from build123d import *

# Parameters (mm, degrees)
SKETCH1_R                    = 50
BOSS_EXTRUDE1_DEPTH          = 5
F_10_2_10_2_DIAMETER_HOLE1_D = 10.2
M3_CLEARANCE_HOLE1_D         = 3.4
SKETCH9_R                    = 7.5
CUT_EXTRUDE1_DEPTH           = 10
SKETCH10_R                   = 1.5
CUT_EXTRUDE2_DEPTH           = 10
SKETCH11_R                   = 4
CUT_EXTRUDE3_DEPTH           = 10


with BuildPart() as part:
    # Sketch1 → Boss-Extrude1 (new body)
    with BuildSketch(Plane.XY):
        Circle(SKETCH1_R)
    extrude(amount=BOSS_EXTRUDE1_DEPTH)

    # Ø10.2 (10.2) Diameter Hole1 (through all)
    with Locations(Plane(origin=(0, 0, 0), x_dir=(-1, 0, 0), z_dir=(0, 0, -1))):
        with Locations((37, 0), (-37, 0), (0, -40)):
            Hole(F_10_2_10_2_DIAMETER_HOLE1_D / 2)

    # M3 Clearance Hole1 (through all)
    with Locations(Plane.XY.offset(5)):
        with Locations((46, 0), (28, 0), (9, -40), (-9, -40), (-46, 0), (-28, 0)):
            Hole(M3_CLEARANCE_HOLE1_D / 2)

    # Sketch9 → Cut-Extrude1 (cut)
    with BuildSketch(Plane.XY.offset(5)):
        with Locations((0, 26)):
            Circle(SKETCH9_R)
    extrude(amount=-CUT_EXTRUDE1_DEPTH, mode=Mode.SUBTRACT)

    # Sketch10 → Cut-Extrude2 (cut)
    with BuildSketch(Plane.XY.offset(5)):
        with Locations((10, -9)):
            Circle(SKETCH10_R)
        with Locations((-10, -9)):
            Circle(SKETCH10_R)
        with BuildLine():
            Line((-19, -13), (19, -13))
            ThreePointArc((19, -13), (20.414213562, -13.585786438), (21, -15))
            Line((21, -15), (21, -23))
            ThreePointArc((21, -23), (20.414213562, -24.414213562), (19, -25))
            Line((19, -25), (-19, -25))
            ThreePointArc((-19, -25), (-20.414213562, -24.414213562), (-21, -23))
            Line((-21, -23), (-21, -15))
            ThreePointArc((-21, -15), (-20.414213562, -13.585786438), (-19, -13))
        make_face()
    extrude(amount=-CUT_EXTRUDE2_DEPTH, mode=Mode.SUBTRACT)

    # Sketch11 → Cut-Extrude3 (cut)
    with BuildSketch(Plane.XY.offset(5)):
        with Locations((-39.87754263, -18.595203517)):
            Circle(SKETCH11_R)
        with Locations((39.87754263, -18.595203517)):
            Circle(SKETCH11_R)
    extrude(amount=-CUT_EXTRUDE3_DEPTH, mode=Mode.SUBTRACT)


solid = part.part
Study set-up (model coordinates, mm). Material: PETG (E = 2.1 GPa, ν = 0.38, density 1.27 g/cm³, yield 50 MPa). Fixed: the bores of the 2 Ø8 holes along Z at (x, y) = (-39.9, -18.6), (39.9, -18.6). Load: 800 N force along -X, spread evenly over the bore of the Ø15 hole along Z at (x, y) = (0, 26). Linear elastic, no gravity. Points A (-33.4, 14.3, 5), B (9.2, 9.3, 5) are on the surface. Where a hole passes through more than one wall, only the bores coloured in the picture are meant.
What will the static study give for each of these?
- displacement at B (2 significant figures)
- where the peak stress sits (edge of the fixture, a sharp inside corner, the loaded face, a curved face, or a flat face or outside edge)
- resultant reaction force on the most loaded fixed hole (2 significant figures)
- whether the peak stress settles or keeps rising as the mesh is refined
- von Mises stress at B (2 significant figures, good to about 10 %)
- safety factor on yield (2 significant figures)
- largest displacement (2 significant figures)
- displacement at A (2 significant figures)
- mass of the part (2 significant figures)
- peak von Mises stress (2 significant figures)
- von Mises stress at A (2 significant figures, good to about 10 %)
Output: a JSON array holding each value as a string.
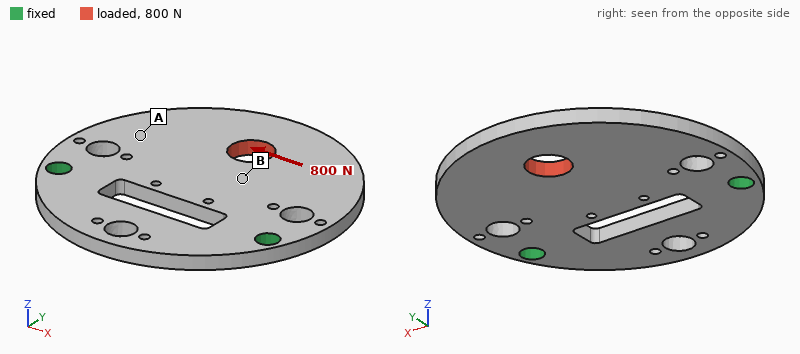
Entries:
["0.13 mm", "a curved face", "580 N", "settles", "4.5 MPa", "3.3", "0.24 mm", "0.15 mm", "43 g", "15 MPa", "1.7 MPa"]
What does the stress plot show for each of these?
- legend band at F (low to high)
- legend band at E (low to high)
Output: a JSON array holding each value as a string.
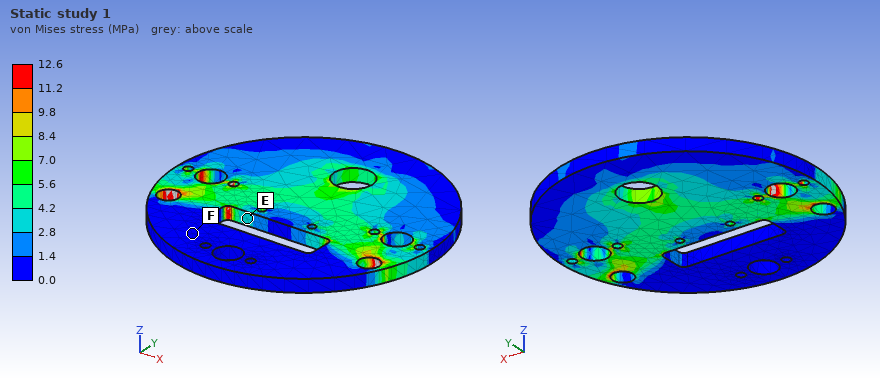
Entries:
["0.0 to 1.4 MPa", "2.8 to 4.2 MPa"]
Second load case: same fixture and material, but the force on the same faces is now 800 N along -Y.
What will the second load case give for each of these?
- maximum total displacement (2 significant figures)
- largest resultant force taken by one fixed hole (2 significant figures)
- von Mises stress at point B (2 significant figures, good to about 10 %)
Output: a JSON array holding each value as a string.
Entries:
["0.14 mm", "420 N", "2.9 MPa"]
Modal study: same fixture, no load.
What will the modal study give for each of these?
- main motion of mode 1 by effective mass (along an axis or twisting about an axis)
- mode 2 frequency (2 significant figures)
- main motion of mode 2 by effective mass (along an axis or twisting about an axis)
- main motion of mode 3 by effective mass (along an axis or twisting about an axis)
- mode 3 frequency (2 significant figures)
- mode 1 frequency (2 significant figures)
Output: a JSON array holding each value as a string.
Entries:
["along Z", "610 Hz", "twisting about Y", "along Z", "760 Hz", "210 Hz"]
